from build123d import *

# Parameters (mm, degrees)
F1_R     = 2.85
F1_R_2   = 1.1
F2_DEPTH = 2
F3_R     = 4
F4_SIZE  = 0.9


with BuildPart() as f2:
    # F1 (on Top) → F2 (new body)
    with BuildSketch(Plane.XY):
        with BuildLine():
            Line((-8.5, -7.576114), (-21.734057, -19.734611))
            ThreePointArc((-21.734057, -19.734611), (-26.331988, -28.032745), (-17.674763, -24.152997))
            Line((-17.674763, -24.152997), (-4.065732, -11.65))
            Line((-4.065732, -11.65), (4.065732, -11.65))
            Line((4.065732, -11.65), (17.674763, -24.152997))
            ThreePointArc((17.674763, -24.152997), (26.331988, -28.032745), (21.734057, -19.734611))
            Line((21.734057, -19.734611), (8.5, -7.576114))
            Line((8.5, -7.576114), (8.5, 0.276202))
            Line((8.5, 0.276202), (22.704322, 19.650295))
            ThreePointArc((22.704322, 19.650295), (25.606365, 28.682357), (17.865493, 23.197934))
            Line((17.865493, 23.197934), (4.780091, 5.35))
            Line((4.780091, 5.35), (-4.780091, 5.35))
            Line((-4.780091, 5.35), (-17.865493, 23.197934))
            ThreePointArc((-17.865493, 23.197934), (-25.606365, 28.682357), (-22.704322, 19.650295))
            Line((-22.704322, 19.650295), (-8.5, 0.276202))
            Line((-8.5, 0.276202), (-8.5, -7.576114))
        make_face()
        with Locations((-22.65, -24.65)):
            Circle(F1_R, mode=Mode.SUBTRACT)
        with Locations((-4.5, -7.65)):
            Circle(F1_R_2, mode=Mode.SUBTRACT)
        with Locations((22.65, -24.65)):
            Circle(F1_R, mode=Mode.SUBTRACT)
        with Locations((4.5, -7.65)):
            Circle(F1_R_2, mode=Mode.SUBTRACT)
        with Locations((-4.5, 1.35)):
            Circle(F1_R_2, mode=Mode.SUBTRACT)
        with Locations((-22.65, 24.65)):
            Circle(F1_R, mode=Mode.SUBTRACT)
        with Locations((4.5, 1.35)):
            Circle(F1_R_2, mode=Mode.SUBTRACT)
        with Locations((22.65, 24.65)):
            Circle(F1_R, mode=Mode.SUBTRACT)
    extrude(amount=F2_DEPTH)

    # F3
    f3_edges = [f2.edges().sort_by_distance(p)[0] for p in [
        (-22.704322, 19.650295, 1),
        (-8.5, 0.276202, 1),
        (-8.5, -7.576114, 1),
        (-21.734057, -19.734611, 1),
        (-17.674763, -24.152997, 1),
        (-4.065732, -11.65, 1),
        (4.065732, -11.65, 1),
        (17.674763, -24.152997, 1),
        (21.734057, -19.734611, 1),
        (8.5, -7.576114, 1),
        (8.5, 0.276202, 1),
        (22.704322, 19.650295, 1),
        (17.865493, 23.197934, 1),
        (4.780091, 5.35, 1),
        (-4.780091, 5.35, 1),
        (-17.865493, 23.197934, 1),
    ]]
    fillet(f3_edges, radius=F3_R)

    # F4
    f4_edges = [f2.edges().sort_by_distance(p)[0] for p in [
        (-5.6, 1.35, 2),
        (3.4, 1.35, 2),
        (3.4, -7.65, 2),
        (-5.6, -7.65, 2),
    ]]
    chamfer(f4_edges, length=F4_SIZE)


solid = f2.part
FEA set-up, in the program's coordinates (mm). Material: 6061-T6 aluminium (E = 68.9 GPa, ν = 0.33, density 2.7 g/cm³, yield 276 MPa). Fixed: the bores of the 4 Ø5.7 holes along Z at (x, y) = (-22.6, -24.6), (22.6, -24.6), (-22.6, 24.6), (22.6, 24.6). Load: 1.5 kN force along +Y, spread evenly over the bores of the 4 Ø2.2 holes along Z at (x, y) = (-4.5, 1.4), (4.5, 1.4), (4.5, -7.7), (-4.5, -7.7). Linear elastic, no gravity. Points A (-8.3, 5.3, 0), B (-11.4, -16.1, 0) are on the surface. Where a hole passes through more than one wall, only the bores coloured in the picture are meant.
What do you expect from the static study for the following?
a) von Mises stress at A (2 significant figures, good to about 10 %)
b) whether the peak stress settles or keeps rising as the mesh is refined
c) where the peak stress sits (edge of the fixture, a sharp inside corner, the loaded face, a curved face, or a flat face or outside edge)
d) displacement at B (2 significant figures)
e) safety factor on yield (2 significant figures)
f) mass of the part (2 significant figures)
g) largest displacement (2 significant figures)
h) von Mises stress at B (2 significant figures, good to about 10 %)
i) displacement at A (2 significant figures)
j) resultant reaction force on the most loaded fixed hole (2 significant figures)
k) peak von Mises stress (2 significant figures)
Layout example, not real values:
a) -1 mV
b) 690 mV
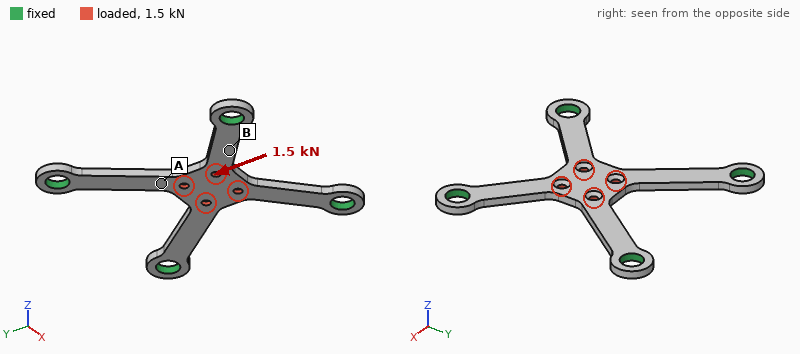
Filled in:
a) 61 MPa
b) settles
c) the loaded face
d) 16 µm
e) 2.2
f) 5.0 g
g) 42 µm
h) 52 MPa
i) 31 µm
j) 490 N
k) 120 MPa
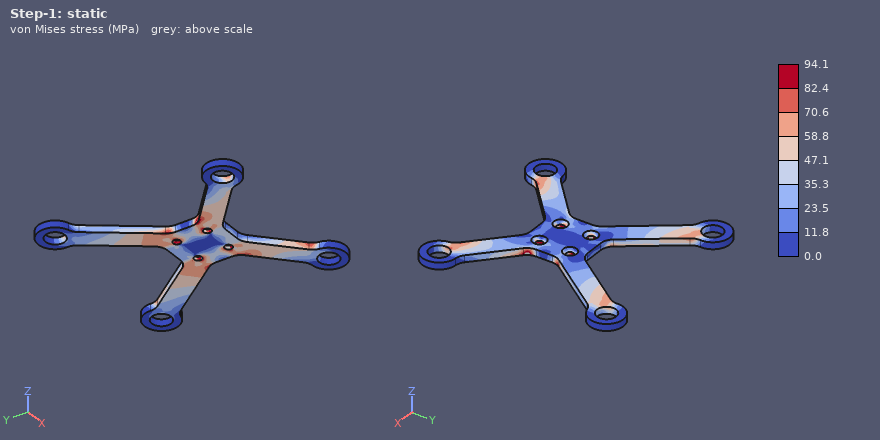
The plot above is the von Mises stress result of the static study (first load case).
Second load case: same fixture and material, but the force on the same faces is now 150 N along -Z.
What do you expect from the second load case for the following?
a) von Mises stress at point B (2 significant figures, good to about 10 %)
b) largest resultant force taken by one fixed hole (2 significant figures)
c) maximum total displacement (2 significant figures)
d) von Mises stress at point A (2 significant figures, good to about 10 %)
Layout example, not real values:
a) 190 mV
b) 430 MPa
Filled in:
a) 13 MPa
b) 45 N
c) 0.22 mm
d) 54 MPa
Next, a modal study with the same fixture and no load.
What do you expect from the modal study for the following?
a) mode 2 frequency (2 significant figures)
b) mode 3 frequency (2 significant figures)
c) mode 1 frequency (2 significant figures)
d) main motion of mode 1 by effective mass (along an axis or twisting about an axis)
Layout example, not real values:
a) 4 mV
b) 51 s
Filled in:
a) 7300 Hz
b) 7800 Hz
c) 3000 Hz
d) along Z
